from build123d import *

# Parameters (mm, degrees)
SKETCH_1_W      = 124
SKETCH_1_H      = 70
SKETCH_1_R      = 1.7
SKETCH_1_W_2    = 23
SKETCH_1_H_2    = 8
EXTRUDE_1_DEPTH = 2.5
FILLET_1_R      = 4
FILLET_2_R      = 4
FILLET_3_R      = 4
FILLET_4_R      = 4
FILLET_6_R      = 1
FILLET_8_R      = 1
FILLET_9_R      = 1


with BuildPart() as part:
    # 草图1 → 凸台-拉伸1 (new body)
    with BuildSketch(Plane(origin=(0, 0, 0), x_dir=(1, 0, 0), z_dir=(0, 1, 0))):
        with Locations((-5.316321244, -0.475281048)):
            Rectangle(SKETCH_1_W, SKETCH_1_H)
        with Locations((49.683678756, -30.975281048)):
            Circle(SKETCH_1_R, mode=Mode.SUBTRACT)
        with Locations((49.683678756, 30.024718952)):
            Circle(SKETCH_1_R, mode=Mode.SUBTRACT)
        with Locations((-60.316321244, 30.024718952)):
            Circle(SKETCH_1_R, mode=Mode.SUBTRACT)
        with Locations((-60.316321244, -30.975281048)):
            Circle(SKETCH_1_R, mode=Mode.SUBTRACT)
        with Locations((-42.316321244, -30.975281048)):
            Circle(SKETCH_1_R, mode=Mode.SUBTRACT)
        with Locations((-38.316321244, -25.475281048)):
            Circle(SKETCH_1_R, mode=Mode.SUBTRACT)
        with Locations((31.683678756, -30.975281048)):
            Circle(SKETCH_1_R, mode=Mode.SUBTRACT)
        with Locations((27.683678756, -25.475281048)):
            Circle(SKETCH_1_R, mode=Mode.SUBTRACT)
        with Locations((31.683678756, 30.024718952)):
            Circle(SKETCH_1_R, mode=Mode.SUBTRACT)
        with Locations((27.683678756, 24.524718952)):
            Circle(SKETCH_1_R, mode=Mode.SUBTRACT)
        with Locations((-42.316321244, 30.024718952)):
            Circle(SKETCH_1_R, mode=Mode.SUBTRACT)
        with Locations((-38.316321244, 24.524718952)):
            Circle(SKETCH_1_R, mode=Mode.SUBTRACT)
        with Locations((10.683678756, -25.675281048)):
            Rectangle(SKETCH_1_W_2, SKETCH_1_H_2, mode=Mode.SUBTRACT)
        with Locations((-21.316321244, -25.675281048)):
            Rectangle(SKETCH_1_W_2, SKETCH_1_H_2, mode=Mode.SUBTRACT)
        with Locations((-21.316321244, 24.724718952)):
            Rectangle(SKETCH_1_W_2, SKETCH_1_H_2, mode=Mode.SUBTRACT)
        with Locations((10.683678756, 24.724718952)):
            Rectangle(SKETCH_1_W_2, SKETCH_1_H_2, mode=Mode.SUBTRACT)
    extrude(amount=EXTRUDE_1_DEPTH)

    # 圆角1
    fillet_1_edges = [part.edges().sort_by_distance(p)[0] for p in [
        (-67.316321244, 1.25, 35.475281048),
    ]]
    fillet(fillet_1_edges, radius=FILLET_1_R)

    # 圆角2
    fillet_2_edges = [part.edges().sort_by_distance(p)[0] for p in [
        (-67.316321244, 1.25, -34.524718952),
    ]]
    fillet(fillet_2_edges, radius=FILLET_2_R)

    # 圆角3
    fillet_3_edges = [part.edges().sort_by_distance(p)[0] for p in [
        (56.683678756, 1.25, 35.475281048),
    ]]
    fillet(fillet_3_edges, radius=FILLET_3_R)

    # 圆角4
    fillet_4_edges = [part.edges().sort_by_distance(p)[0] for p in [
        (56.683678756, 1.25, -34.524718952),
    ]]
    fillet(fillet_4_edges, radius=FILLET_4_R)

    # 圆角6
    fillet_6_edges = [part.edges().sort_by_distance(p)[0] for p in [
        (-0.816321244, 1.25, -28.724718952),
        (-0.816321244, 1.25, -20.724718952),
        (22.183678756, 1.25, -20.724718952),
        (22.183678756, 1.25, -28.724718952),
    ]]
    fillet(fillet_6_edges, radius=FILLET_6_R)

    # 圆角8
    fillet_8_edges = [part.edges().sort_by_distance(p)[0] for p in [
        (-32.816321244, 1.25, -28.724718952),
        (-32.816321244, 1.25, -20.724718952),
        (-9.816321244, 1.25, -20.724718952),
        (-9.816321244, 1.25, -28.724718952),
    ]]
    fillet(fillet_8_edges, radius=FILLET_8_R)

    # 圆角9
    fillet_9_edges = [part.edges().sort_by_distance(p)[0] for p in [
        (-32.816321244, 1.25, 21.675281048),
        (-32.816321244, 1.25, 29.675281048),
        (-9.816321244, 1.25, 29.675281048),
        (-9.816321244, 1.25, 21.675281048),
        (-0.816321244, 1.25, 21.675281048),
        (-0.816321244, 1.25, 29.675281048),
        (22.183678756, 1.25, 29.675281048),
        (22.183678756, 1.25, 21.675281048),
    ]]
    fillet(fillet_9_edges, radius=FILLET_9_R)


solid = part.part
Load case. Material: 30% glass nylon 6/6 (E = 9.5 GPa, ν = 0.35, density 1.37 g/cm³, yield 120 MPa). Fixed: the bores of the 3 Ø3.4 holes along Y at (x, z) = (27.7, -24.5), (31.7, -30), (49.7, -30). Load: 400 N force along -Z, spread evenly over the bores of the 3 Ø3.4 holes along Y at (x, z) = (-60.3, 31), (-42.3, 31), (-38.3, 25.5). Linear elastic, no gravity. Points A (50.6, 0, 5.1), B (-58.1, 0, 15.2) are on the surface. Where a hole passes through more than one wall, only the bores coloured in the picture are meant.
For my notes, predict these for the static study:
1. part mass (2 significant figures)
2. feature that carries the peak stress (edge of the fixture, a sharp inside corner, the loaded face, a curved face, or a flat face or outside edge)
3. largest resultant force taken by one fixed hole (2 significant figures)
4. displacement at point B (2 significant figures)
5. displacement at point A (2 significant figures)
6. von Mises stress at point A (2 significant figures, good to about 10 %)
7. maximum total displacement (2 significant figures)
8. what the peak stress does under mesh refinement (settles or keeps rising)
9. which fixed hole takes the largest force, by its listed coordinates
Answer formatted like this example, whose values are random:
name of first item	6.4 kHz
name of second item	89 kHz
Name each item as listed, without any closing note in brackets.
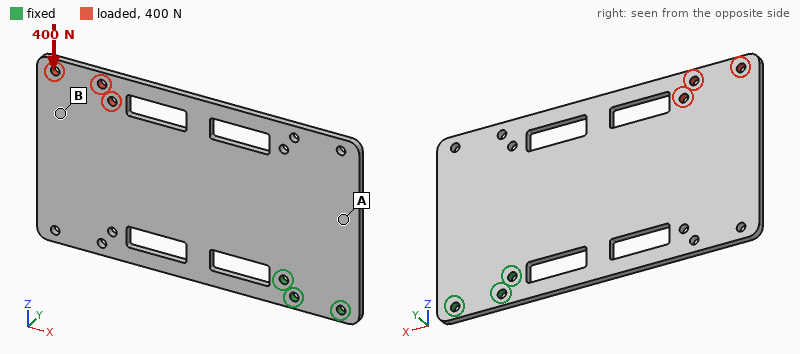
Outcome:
part mass	27 g
feature that carries the peak stress	edge of the fixture
largest resultant force taken by one fixed hole	1.5 kN
displacement at point B	1.1 mm
displacement at point A	0.26 mm
von Mises stress at point A	13 MPa
maximum total displacement	1.3 mm
what the peak stress does under mesh refinement	keeps rising
which fixed hole takes the largest force, by its listed coordinates	(27.7, -24.5)
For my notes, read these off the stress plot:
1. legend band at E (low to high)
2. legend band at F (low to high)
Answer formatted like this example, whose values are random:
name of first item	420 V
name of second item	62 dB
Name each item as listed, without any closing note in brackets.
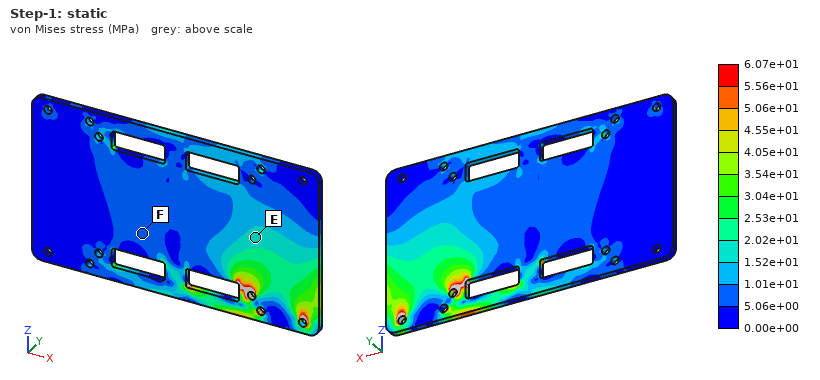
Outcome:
legend band at E	1.52e+01 to 2.02e+01 MPa
legend band at F	5.06e+00 to 1.01e+01 MPa
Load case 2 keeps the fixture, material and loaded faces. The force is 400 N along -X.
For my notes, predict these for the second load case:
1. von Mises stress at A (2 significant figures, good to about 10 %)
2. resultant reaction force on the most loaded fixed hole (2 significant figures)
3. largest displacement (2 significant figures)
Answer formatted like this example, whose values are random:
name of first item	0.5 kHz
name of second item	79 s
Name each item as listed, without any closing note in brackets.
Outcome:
von Mises stress at A	8.6 MPa
resultant reaction force on the most loaded fixed hole	940 N
largest displacement	0.84 mm
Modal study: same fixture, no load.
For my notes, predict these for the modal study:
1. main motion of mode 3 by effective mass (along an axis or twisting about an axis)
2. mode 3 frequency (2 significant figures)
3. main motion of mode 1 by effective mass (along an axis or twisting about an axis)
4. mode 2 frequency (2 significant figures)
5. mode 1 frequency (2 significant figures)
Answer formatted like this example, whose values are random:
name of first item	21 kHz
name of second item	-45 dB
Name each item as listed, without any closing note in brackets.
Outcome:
main motion of mode 3 by effective mass	along Y
mode 3 frequency	420 Hz
main motion of mode 1 by effective mass	along Y
mode 2 frequency	210 Hz
mode 1 frequency	85 Hz
